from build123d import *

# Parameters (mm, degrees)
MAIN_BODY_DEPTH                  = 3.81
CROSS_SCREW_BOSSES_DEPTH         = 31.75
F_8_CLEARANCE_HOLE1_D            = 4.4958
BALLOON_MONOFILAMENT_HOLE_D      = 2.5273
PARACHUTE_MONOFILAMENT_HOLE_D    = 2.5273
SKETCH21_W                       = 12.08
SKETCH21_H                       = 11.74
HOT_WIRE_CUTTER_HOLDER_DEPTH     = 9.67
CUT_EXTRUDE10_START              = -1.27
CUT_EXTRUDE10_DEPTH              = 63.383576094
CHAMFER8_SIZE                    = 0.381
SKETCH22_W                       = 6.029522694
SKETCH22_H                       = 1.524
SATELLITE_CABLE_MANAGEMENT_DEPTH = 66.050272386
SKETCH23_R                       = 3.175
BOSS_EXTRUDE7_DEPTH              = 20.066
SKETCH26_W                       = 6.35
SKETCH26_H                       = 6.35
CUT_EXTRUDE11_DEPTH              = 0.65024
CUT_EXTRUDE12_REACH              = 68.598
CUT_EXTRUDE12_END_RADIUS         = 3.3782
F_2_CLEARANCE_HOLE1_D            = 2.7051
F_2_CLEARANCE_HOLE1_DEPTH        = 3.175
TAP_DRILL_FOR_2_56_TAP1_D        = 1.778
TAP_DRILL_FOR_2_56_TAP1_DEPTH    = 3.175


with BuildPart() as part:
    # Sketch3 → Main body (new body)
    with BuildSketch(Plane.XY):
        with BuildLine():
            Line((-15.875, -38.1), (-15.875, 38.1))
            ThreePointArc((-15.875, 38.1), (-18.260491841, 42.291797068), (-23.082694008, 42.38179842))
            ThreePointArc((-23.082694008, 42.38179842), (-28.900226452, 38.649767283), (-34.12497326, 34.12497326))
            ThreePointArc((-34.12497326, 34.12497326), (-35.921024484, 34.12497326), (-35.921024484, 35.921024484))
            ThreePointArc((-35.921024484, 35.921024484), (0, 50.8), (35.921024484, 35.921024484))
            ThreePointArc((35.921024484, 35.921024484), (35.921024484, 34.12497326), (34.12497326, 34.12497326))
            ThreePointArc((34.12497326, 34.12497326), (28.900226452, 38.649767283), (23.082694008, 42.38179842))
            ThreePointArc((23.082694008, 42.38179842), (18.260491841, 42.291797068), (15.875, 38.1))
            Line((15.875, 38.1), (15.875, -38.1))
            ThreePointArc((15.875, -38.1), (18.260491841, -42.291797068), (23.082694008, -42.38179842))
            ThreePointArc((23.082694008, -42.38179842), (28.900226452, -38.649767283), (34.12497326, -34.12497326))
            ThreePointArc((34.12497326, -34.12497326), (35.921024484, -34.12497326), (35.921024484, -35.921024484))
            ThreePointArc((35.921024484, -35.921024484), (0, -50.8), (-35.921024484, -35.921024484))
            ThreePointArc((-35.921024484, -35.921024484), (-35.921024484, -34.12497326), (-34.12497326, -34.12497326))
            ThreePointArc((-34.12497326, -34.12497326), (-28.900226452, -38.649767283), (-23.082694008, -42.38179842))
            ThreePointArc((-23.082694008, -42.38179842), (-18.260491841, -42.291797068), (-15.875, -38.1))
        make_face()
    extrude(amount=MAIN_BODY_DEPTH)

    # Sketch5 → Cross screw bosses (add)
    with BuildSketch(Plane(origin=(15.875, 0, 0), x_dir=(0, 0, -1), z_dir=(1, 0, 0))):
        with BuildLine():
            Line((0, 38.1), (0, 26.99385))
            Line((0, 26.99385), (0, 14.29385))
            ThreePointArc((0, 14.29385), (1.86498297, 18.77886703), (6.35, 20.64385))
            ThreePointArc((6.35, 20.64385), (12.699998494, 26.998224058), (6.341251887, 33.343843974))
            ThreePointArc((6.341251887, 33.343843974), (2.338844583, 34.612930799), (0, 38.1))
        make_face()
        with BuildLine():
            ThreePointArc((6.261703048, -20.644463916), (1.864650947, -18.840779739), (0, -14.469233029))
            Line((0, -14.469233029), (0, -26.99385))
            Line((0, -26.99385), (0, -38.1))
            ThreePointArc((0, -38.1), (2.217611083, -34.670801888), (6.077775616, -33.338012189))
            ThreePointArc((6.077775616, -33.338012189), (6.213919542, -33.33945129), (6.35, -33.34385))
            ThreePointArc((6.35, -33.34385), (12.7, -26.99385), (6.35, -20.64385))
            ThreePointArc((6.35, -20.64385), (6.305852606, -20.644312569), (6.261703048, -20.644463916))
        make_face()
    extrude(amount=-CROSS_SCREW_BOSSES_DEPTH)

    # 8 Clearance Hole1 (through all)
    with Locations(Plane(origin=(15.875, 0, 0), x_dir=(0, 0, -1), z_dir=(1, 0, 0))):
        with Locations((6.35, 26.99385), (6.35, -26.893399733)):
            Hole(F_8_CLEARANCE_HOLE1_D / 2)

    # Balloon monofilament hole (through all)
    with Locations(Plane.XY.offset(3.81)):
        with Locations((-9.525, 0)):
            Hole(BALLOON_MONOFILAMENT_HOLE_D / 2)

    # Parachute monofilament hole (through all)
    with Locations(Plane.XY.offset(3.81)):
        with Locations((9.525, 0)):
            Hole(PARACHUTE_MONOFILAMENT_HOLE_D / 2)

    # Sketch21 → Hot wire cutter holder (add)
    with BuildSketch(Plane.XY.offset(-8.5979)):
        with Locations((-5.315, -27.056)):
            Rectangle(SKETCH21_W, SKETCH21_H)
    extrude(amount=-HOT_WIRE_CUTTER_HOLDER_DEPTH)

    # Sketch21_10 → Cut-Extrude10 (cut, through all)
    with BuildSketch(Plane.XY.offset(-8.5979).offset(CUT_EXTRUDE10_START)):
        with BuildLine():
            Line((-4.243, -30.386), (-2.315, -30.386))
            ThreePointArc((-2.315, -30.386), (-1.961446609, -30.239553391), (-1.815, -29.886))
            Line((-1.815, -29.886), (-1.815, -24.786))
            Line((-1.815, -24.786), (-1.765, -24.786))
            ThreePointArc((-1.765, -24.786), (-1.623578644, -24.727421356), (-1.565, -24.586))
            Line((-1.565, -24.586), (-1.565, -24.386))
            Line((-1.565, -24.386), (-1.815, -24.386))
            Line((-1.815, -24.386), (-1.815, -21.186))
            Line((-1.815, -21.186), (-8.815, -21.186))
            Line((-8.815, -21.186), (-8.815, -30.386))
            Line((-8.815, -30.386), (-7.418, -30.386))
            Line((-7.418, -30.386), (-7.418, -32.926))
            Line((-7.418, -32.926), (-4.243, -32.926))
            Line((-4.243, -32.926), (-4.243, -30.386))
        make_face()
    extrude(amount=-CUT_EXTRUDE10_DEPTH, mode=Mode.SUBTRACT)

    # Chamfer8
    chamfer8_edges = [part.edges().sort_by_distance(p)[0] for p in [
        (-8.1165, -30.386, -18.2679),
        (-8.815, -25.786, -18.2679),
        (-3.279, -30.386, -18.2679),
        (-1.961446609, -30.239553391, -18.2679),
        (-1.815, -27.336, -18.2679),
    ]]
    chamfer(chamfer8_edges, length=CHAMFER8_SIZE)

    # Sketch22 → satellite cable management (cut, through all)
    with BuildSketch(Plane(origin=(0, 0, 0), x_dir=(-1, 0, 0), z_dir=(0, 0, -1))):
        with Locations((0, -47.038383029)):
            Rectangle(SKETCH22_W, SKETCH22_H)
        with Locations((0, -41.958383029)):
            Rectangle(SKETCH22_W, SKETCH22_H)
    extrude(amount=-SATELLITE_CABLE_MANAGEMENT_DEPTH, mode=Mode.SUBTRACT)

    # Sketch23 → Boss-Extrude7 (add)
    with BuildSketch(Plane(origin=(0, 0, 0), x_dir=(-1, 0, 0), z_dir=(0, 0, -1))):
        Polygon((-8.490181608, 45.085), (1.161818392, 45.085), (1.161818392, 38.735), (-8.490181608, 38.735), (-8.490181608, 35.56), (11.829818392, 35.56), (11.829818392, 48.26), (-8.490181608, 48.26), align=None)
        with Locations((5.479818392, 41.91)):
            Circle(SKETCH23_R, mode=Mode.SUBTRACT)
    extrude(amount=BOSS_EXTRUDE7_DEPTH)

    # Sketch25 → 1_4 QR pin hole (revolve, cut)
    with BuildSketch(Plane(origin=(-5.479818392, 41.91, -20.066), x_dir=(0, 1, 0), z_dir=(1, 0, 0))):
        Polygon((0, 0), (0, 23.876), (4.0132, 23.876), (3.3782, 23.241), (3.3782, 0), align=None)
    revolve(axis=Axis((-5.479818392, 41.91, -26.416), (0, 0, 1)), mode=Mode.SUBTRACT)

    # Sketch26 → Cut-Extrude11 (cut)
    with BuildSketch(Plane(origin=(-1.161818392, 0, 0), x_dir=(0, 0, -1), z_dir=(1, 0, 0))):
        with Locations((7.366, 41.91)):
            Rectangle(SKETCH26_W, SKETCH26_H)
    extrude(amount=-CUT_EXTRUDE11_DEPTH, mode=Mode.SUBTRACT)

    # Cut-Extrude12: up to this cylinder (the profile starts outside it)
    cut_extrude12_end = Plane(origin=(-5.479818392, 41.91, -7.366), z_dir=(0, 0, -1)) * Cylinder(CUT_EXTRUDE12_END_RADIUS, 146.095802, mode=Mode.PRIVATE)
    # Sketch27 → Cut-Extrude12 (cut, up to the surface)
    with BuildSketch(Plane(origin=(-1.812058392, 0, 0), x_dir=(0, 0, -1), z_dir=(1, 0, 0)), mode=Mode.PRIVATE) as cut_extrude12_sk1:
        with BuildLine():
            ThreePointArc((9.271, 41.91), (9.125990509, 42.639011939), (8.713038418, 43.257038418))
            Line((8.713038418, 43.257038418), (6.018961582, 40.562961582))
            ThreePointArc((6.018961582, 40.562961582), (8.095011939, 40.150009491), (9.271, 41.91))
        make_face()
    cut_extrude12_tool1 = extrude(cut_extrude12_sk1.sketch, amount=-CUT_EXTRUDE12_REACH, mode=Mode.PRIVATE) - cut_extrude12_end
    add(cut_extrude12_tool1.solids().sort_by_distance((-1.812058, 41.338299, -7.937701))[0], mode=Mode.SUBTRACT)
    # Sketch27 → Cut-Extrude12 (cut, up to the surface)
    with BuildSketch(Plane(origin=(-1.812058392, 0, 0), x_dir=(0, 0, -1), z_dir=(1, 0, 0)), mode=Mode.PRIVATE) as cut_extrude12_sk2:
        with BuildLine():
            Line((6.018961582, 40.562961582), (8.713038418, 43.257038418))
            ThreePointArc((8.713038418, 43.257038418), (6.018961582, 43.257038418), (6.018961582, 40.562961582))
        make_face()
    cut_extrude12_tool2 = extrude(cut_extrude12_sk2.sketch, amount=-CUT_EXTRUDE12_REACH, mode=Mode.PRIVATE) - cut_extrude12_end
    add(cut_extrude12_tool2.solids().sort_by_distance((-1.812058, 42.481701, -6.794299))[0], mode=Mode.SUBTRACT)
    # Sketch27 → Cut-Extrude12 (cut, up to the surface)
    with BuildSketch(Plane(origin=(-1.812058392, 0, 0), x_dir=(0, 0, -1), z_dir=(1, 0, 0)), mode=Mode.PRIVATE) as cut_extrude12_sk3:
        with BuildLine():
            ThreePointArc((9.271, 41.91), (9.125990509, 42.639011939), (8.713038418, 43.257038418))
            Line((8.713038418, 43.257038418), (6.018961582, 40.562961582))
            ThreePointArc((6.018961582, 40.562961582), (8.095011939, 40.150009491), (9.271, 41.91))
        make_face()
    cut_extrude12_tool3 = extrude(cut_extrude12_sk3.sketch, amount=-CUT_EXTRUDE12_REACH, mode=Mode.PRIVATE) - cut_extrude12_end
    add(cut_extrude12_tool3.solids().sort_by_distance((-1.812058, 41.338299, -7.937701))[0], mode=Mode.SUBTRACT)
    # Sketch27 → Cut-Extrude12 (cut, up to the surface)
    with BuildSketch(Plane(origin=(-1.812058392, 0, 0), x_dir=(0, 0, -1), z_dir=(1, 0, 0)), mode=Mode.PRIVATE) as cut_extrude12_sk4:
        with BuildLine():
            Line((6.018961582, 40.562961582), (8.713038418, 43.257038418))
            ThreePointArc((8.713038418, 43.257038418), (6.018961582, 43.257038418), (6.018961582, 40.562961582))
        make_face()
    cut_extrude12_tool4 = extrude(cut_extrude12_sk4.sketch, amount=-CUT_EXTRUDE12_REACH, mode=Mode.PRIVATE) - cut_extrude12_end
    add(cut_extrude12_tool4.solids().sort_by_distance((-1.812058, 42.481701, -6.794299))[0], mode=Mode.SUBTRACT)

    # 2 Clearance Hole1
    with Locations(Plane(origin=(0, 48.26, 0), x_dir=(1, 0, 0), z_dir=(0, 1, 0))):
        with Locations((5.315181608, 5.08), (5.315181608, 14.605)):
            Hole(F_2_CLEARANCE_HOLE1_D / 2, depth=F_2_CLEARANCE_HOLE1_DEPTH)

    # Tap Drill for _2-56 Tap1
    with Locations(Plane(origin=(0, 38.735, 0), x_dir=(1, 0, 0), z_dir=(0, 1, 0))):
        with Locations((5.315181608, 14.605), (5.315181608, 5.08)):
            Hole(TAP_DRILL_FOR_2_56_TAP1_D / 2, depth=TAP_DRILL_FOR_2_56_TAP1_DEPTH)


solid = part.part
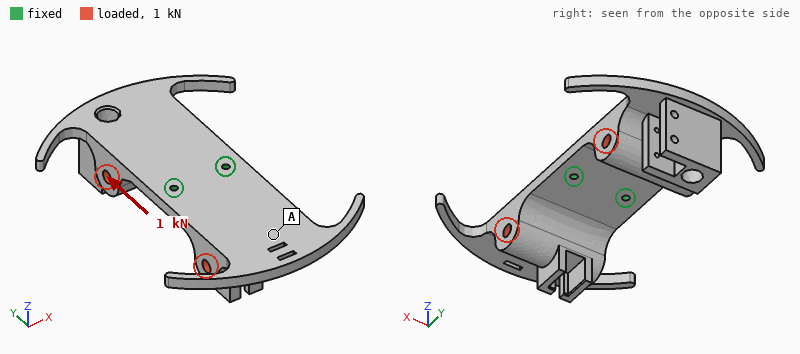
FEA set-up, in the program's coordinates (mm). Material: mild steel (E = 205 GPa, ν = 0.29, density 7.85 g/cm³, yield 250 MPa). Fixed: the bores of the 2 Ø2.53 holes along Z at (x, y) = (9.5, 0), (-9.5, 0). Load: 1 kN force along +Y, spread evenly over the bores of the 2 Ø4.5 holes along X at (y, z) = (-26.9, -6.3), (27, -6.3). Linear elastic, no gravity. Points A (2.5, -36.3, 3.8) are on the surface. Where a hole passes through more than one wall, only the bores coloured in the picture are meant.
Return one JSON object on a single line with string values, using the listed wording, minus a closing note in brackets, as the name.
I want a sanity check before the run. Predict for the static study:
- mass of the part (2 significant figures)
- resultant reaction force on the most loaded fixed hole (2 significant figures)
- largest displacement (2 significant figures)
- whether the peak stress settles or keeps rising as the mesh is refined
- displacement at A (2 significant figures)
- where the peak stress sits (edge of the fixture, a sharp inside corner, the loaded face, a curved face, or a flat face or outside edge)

{"mass of the part": "200 g", "resultant reaction force on the most loaded fixed hole": "500 N", "largest displacement": "0.13 mm", "whether the peak stress settles or keeps rising as the mesh is refined": "keeps rising", "displacement at A": "0.078 mm", "where the peak stress sits": "edge of the fixture"}
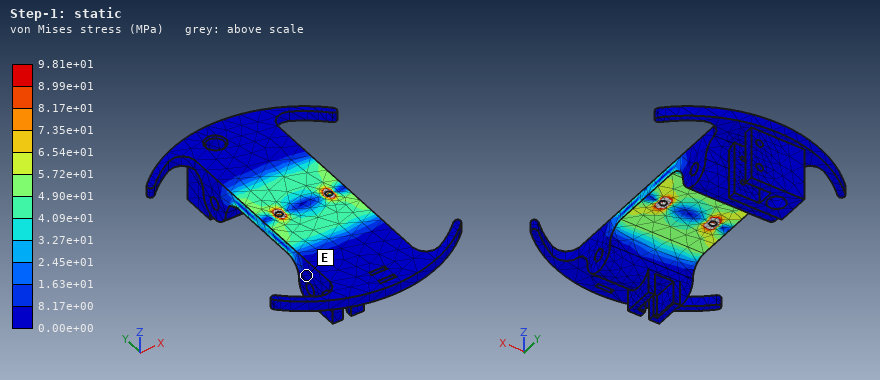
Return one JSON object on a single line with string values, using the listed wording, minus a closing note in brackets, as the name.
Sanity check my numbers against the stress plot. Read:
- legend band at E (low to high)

{"legend band at E": "0.00e+00 to 8.17e+00 MPa"}
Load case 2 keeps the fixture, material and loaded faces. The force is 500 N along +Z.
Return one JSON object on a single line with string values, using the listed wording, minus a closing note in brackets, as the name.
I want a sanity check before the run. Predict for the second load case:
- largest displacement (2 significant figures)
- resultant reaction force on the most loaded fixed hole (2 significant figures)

{"largest displacement": "0.12 mm", "resultant reaction force on the most loaded fixed hole": "250 N"}
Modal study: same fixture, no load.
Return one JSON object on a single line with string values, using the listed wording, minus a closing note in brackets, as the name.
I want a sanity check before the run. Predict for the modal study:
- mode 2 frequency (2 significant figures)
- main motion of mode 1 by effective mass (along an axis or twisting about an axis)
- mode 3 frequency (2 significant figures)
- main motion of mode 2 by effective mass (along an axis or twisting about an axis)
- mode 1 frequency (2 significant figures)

{"mode 2 frequency": "960 Hz", "main motion of mode 1 by effective mass": "along Z", "mode 3 frequency": "2700 Hz", "main motion of mode 2 by effective mass": "along Z", "mode 1 frequency": "720 Hz"}
